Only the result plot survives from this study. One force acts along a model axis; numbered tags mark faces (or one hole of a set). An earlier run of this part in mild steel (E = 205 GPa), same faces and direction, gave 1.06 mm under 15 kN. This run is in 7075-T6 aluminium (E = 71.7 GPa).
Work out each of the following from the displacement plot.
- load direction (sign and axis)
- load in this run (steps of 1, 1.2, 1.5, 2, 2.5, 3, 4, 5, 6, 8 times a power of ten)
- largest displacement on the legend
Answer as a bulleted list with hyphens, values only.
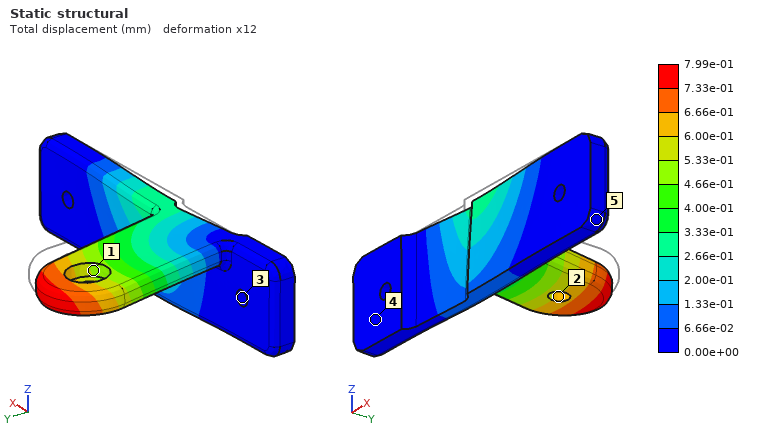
- -X
- 4 kN
- 7.99e-01 mm
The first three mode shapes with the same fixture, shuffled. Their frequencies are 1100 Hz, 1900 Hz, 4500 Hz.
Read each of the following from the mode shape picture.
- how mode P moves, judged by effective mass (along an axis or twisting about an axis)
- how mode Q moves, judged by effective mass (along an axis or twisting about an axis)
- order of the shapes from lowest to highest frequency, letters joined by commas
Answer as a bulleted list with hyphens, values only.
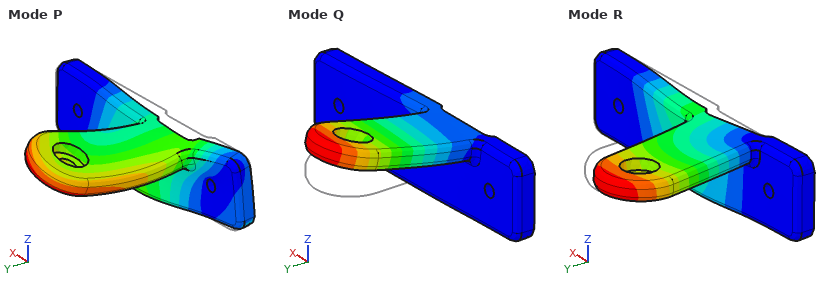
- along Y
- along Z
- Q, R, P
